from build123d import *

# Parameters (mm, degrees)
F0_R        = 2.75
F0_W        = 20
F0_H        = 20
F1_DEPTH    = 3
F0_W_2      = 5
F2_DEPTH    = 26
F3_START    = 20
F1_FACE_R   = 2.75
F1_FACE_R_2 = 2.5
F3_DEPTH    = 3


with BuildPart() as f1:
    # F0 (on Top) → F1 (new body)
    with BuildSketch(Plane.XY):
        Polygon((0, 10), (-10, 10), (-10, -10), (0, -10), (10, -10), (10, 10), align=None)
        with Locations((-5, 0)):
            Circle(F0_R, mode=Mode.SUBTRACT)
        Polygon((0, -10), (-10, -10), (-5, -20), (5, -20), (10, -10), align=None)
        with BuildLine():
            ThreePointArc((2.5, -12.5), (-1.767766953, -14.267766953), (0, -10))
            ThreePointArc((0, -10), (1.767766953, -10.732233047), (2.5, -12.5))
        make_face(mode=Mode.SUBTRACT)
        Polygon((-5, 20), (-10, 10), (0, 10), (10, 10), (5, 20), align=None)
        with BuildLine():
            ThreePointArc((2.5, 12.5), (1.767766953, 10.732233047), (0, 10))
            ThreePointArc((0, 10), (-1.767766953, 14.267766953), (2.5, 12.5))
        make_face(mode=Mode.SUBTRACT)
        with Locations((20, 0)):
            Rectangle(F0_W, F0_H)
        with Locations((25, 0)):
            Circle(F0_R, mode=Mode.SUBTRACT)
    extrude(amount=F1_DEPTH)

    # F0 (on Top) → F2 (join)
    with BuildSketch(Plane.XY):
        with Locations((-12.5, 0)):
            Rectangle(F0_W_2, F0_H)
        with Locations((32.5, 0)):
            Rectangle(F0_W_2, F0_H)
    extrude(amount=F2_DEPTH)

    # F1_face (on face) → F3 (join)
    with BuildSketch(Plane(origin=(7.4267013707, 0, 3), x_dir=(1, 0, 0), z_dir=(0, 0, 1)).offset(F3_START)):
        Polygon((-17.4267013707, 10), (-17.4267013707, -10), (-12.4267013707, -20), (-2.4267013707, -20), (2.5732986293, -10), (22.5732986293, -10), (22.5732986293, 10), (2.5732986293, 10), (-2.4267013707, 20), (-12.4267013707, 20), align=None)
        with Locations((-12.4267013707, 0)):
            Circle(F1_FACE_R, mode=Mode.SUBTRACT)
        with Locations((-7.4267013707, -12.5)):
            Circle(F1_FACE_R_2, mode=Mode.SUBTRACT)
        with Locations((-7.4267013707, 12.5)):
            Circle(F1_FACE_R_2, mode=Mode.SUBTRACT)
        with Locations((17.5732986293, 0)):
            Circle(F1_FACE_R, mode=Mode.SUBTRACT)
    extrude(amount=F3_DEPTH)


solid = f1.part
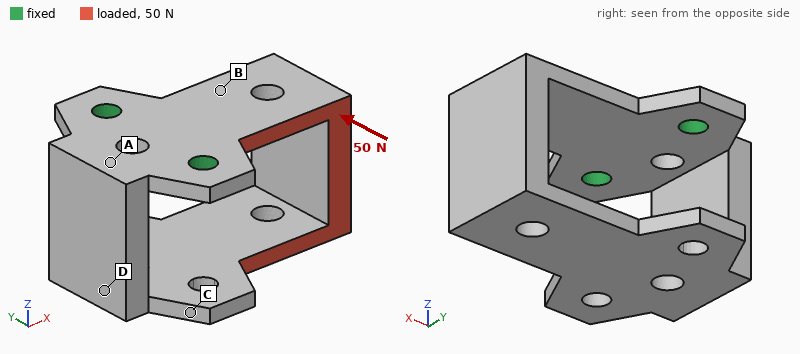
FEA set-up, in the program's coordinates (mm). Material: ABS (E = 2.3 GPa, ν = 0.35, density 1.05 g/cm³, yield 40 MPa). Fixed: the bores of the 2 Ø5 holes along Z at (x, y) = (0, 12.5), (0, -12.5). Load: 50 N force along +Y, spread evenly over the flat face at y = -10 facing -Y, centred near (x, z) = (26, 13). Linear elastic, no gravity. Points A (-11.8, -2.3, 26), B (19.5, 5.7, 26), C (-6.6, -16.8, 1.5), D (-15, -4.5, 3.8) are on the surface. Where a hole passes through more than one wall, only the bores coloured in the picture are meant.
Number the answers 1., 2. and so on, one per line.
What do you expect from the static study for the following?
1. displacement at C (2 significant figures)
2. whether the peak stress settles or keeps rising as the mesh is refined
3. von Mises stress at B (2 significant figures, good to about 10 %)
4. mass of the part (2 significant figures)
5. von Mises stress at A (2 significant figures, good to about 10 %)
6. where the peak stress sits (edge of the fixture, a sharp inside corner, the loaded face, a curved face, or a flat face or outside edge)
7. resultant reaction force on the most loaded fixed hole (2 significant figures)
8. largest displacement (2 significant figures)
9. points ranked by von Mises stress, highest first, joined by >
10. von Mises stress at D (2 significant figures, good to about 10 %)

1. 0.33 mm
2. keeps rising
3. 4.6 MPa
4. 12 g
5. 3.7 MPa
6. a sharp inside corner
7. 65 N
8. 0.75 mm
9. B > A > D > C
10. 1.5 MPa
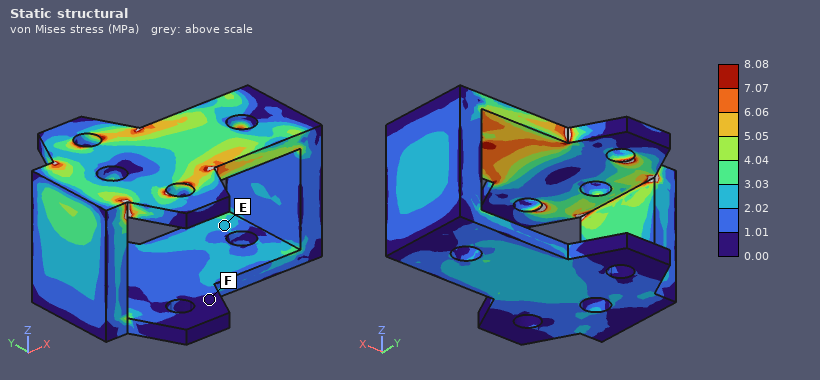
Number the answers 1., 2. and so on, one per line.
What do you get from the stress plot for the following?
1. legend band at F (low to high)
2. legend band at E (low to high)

1. 0.00 to 1.01 MPa
2. 2.02 to 3.03 MPa
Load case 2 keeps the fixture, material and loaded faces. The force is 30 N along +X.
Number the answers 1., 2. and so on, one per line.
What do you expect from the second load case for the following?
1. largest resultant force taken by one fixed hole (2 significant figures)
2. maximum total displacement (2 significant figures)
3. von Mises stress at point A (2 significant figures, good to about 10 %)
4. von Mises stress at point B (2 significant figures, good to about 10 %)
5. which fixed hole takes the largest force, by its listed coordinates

1. 27 N
2. 0.64 mm
3. 2.1 MPa
4. 2.4 MPa
5. (0, -12.5)
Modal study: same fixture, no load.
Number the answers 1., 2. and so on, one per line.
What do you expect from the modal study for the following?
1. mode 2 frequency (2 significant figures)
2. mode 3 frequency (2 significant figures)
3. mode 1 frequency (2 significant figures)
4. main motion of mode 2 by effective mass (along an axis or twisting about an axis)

1. 570 Hz
2. 750 Hz
3. 300 Hz
4. along Y
